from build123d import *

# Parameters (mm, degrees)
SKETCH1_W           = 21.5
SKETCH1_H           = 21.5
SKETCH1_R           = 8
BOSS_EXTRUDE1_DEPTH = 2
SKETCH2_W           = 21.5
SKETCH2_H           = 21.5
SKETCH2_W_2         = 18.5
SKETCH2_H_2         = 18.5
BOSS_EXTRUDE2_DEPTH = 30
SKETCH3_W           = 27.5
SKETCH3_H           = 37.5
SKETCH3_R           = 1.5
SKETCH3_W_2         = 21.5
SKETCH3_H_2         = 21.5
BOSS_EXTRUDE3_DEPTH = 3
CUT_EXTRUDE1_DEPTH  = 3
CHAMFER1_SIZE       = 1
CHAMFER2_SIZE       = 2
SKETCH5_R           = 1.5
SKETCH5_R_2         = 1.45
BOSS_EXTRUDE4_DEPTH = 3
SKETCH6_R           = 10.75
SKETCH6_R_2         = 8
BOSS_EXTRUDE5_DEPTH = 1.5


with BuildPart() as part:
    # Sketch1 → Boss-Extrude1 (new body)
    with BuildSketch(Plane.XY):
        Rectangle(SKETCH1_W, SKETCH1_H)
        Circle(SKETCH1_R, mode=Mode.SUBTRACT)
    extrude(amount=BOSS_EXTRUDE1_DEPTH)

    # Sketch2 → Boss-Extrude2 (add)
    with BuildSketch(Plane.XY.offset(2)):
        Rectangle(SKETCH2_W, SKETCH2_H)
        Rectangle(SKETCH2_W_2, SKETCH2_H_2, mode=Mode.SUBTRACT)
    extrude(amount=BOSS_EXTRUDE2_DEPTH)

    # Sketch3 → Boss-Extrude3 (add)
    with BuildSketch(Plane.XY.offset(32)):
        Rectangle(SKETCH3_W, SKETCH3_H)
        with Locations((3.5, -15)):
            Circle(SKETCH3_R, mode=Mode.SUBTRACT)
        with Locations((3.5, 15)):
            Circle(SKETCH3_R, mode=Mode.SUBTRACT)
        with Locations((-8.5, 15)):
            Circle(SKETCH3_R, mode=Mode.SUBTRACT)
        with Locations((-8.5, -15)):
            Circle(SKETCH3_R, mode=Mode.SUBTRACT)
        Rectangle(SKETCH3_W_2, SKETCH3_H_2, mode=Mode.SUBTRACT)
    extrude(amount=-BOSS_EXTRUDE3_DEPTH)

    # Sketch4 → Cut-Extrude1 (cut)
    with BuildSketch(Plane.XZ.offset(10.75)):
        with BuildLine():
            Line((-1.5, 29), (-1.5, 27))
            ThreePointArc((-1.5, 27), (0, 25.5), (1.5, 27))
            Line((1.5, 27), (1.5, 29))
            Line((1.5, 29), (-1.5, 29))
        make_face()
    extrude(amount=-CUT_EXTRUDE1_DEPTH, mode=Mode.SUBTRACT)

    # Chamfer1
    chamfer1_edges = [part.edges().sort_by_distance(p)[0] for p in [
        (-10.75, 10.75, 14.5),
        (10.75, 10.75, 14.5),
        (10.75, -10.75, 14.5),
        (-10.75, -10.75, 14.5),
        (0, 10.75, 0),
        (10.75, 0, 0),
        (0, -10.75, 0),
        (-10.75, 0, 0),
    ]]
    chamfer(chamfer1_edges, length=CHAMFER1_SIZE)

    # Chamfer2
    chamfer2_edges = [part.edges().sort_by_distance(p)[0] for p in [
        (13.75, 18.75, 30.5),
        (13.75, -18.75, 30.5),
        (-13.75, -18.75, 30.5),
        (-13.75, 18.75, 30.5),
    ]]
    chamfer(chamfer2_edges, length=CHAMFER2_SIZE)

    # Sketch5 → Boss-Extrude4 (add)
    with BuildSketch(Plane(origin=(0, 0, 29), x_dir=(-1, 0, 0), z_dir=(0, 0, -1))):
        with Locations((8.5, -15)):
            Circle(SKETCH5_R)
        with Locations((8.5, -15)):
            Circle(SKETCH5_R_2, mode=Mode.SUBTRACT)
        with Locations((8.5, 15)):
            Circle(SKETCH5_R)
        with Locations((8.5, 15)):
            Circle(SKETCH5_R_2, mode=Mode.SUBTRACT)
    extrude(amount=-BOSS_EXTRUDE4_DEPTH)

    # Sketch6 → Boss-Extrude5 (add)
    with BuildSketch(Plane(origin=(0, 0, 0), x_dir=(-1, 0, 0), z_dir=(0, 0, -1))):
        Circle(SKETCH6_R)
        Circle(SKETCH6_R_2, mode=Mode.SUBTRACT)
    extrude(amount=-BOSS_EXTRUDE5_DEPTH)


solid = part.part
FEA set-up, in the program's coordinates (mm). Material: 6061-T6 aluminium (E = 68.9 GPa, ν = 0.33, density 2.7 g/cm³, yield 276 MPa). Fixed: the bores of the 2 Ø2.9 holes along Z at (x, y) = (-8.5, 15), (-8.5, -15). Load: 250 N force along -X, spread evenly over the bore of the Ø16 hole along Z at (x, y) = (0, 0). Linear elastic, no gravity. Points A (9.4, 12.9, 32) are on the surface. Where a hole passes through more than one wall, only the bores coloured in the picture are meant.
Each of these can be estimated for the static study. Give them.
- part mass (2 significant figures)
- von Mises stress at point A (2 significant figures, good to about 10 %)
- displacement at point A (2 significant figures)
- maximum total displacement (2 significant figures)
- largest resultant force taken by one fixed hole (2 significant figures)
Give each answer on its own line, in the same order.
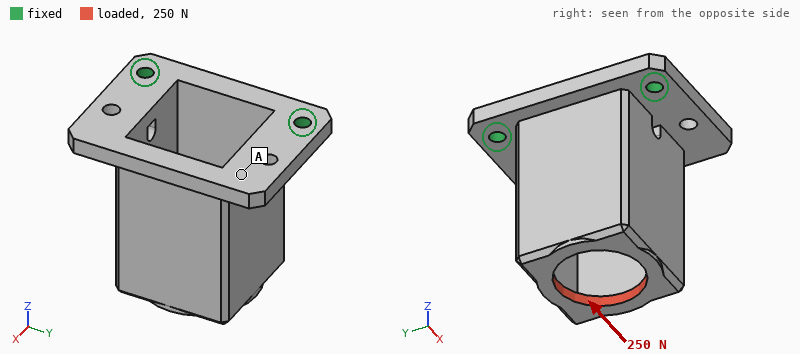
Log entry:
15 g
24 MPa
0.12 mm
0.27 mm
130 N
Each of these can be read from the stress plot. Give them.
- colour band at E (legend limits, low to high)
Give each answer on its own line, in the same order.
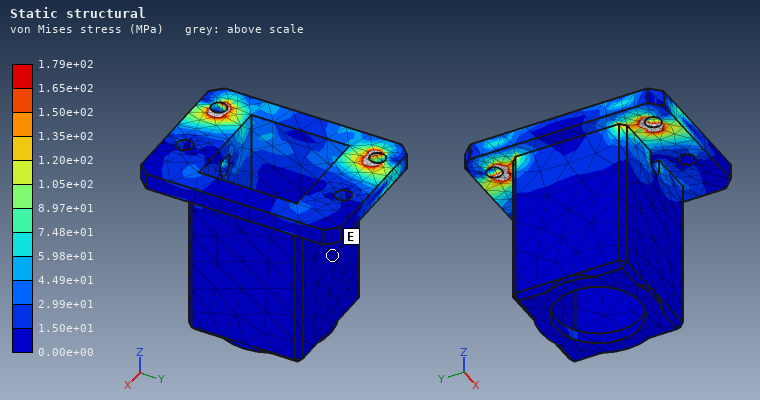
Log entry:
0.00e+00 to 1.50e+01 MPa
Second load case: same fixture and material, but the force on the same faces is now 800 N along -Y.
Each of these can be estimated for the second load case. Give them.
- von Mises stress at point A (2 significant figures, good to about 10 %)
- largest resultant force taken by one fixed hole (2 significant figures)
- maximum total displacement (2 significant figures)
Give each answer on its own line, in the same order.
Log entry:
29 MPa
1.1 kN
0.12 mm
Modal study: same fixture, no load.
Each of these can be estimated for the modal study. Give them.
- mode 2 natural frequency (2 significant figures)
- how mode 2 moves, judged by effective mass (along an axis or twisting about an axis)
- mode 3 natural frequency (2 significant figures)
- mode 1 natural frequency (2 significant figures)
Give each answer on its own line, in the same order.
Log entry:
6100 Hz
along Y
9000 Hz
2100 Hz
